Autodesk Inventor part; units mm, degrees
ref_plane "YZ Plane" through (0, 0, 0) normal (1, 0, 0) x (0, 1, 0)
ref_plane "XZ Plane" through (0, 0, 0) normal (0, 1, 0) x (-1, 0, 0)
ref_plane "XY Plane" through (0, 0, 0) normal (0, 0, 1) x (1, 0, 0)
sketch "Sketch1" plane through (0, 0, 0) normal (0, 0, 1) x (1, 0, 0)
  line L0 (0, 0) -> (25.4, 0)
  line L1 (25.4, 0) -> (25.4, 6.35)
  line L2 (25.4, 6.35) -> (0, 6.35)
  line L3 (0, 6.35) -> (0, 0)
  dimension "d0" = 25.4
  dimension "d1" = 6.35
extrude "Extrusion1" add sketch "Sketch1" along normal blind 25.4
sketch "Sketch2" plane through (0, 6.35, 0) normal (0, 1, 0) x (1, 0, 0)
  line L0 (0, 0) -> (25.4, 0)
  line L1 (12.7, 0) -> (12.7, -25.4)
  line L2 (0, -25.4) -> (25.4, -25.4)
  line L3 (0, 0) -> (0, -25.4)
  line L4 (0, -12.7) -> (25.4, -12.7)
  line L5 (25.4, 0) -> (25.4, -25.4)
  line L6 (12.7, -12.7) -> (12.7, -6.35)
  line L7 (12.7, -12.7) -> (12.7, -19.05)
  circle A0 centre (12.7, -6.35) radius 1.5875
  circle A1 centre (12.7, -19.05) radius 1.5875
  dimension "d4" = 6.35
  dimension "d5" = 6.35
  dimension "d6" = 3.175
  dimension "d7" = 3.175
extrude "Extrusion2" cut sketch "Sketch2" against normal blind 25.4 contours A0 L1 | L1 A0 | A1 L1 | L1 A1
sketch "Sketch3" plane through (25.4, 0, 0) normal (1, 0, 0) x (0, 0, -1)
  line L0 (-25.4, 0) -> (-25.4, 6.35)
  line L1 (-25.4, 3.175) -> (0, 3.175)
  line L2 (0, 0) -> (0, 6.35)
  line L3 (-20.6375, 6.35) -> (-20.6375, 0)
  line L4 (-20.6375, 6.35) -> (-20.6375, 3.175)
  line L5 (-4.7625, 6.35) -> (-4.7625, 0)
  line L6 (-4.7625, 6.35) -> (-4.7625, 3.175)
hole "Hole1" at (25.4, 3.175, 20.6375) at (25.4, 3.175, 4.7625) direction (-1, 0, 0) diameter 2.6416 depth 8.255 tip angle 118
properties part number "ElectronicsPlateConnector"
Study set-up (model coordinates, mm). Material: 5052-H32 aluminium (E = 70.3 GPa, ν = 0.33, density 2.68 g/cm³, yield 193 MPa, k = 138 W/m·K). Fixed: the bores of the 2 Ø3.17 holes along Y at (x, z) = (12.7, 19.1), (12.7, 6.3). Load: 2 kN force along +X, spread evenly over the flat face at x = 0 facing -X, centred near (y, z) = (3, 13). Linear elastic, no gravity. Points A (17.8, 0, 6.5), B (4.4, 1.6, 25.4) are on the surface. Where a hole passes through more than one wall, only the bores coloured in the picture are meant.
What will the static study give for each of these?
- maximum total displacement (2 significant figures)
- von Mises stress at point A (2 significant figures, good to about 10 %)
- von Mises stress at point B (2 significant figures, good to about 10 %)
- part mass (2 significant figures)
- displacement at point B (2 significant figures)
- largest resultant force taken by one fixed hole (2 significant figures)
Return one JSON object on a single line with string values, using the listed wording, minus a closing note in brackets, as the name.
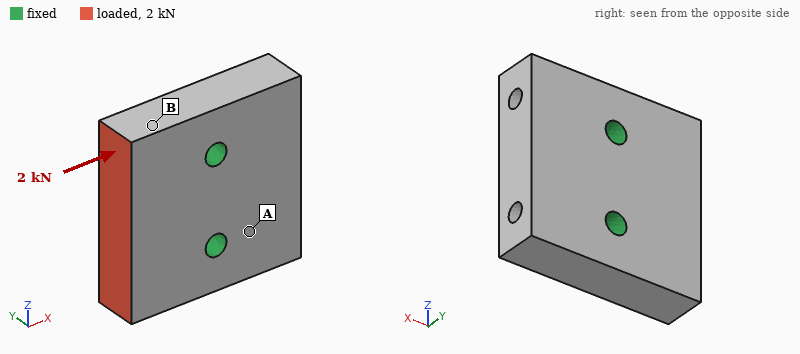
{"maximum total displacement": "2.9 µm", "von Mises stress at point A": "4.1 MPa", "von Mises stress at point B": "11 MPa", "part mass": "10 g", "displacement at point B": "2.2 µm", "largest resultant force taken by one fixed hole": "1.0 kN"}
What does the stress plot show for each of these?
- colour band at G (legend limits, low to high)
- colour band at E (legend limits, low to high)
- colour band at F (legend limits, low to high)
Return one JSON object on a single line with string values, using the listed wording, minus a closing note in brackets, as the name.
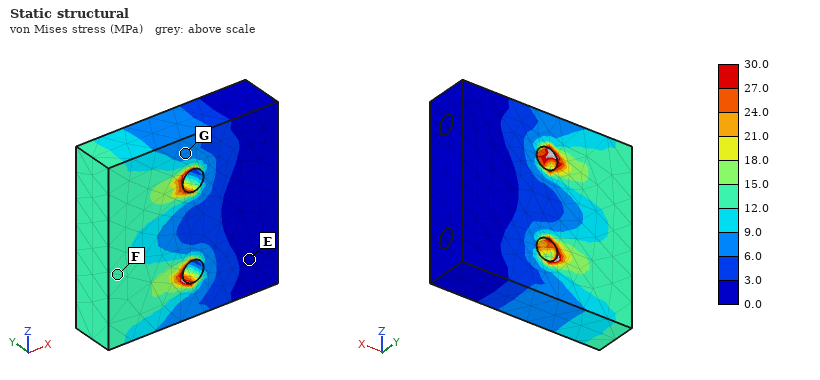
{"colour band at G": "6.0 to 9.0 MPa", "colour band at E": "0.0 to 3.0 MPa", "colour band at F": "12.0 to 15.0 MPa"}
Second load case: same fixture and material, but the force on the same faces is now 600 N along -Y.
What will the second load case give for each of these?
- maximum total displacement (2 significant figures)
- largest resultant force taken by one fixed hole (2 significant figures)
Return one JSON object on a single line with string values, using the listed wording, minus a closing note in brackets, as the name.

{"maximum total displacement": "14 µm", "largest resultant force taken by one fixed hole": "300 N"}
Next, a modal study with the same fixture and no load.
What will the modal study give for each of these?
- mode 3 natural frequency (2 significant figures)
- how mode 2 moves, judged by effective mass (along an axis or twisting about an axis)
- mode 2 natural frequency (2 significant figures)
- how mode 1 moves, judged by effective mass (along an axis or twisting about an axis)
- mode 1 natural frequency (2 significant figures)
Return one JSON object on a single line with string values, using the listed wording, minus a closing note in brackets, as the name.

{"mode 3 natural frequency": "36 kHz", "how mode 2 moves, judged by effective mass": "along Y", "mode 2 natural frequency": "31 kHz", "how mode 1 moves, judged by effective mass": "twisting about Z", "mode 1 natural frequency": "25 kHz"}
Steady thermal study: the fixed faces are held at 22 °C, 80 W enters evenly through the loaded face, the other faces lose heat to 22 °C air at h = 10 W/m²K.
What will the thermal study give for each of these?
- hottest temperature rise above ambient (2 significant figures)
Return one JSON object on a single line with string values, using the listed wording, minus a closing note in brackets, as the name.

{"hottest temperature rise above ambient": "46 K"}
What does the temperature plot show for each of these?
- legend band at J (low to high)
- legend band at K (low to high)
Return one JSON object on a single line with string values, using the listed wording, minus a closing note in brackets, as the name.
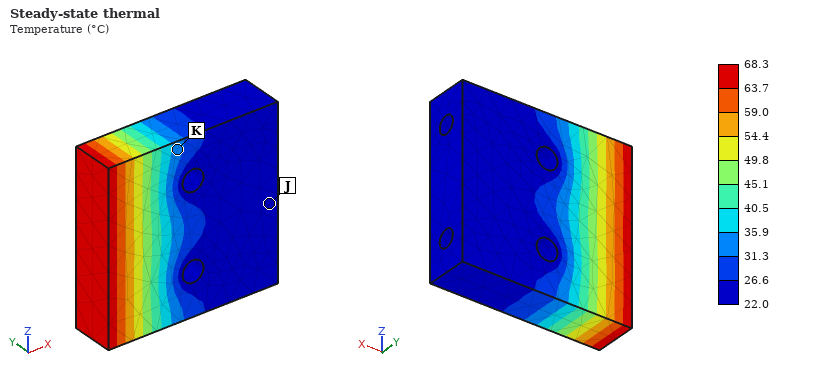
{"legend band at J": "22.0 to 26.6 °C", "legend band at K": "31.3 to 35.9 °C"}
